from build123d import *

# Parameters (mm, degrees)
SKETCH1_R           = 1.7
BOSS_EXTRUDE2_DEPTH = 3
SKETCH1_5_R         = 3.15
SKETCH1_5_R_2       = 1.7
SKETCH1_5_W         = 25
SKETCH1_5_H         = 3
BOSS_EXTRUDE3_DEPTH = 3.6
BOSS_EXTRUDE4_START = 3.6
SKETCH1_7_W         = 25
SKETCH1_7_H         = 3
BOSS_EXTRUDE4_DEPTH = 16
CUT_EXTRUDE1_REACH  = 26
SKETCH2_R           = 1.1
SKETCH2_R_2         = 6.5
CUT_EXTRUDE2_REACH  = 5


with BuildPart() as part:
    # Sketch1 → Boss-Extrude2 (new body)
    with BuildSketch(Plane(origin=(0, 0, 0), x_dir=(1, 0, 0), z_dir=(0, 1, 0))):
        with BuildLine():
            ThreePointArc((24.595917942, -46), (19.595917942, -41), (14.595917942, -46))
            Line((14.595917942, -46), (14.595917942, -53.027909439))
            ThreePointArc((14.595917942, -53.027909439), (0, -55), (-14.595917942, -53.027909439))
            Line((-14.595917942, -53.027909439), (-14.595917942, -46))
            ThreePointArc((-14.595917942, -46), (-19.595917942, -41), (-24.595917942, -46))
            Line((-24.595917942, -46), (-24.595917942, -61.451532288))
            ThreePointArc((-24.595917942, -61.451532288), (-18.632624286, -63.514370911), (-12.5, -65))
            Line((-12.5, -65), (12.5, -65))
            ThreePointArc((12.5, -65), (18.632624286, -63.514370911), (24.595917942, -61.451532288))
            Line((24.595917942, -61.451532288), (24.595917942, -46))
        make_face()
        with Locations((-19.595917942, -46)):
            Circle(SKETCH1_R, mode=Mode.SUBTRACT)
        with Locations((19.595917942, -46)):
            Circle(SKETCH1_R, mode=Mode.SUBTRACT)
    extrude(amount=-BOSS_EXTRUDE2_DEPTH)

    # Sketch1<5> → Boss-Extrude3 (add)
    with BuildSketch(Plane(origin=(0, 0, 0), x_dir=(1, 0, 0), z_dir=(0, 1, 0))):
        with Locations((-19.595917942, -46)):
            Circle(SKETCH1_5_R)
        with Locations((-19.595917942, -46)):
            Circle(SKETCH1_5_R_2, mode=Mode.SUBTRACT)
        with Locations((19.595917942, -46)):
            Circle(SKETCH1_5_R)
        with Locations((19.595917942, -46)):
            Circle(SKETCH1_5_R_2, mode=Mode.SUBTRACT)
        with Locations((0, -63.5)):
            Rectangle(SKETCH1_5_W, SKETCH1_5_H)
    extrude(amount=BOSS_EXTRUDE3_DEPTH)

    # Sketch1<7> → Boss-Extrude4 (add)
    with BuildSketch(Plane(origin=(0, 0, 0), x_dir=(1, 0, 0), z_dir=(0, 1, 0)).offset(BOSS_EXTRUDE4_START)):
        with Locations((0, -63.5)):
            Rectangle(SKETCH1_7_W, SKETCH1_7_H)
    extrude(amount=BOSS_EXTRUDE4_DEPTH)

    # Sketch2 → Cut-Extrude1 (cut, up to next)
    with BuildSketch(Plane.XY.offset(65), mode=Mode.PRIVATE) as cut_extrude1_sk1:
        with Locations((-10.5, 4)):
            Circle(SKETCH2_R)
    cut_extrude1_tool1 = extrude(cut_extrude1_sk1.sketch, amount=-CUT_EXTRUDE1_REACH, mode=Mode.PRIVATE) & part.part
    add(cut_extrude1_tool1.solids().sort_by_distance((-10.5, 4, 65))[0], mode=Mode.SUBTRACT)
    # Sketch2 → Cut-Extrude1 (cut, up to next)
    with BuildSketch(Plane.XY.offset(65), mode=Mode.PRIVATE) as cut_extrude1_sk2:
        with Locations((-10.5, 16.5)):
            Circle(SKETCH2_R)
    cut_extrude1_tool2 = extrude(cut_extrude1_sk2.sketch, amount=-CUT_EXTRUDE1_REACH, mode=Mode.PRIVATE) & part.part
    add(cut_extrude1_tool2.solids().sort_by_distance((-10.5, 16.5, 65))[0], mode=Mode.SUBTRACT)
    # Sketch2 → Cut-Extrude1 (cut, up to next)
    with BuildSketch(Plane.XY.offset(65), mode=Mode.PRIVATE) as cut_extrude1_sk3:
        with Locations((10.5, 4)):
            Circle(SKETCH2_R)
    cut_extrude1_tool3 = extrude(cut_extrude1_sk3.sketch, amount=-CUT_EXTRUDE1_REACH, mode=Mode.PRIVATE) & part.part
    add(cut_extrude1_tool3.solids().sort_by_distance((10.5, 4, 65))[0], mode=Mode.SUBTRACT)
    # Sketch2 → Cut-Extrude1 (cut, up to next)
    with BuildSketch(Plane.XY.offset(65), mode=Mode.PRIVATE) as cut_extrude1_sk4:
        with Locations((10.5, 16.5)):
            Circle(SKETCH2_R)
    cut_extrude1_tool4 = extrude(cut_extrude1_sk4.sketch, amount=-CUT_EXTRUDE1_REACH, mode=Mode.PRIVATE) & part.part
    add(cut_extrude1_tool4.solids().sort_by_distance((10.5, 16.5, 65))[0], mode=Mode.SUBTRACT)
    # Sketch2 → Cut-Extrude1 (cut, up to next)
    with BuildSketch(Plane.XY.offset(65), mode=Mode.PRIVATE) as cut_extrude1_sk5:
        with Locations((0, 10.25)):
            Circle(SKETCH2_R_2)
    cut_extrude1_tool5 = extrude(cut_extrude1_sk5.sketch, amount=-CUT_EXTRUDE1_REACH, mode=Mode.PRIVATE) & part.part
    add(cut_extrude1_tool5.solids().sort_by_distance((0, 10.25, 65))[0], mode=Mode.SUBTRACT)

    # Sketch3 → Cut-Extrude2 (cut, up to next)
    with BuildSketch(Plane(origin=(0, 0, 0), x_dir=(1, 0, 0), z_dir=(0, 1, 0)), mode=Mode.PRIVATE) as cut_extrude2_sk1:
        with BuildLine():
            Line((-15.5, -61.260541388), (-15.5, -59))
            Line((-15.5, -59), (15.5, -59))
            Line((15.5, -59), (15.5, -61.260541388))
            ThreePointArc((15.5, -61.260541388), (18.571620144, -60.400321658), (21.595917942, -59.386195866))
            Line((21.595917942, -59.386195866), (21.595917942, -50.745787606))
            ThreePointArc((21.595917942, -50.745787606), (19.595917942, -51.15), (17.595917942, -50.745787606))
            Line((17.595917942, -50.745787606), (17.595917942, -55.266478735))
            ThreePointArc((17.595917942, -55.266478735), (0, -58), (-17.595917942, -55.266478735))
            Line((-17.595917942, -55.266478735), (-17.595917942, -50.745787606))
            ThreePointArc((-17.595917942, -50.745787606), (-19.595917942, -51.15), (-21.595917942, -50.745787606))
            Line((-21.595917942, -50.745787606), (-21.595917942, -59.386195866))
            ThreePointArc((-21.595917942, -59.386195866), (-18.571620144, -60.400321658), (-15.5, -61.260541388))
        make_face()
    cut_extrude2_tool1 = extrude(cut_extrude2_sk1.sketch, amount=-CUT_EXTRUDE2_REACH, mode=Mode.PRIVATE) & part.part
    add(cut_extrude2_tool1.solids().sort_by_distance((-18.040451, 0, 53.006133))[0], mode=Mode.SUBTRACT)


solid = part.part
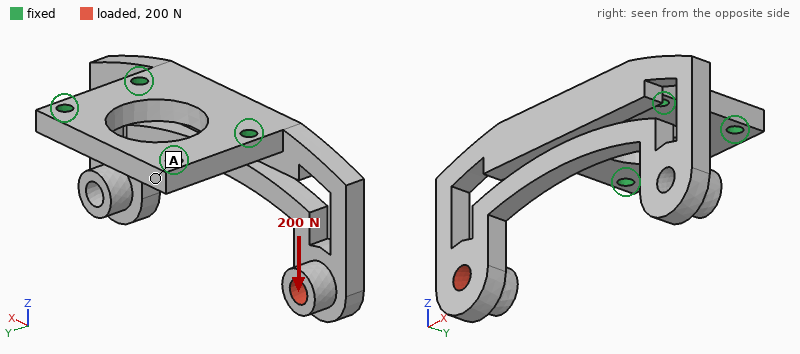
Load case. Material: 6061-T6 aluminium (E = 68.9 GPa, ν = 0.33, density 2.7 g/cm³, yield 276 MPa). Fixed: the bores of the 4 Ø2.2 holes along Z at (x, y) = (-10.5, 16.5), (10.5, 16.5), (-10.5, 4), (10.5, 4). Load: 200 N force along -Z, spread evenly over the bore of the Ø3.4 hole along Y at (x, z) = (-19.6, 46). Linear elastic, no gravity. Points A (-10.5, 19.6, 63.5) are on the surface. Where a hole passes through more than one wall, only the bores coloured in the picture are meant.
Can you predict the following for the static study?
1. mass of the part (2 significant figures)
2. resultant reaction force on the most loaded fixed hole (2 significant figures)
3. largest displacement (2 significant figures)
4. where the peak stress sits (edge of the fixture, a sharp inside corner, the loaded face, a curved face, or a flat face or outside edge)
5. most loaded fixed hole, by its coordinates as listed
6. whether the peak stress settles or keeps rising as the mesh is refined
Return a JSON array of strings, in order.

["7.8 g", "280 N", "0.27 mm", "edge of the fixture", "(-10.5, 4)", "keeps rising"]
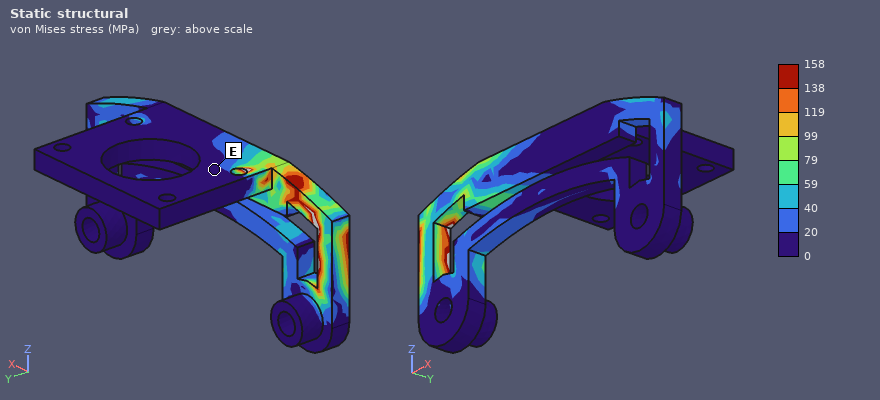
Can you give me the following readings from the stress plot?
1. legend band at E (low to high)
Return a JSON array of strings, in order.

["0 to 20 MPa"]
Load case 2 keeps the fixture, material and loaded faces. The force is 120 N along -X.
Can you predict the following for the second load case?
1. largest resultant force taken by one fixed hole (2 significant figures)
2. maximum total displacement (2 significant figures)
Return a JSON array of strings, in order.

["110 N", "0.39 mm"]
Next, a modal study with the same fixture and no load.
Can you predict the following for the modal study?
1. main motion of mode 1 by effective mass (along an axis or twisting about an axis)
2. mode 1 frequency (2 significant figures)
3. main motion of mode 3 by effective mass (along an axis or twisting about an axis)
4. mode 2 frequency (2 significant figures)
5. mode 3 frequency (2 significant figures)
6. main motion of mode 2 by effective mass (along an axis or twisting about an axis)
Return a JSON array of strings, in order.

["along Y", "1500 Hz", "along X", "2000 Hz", "2700 Hz", "twisting about Z"]
